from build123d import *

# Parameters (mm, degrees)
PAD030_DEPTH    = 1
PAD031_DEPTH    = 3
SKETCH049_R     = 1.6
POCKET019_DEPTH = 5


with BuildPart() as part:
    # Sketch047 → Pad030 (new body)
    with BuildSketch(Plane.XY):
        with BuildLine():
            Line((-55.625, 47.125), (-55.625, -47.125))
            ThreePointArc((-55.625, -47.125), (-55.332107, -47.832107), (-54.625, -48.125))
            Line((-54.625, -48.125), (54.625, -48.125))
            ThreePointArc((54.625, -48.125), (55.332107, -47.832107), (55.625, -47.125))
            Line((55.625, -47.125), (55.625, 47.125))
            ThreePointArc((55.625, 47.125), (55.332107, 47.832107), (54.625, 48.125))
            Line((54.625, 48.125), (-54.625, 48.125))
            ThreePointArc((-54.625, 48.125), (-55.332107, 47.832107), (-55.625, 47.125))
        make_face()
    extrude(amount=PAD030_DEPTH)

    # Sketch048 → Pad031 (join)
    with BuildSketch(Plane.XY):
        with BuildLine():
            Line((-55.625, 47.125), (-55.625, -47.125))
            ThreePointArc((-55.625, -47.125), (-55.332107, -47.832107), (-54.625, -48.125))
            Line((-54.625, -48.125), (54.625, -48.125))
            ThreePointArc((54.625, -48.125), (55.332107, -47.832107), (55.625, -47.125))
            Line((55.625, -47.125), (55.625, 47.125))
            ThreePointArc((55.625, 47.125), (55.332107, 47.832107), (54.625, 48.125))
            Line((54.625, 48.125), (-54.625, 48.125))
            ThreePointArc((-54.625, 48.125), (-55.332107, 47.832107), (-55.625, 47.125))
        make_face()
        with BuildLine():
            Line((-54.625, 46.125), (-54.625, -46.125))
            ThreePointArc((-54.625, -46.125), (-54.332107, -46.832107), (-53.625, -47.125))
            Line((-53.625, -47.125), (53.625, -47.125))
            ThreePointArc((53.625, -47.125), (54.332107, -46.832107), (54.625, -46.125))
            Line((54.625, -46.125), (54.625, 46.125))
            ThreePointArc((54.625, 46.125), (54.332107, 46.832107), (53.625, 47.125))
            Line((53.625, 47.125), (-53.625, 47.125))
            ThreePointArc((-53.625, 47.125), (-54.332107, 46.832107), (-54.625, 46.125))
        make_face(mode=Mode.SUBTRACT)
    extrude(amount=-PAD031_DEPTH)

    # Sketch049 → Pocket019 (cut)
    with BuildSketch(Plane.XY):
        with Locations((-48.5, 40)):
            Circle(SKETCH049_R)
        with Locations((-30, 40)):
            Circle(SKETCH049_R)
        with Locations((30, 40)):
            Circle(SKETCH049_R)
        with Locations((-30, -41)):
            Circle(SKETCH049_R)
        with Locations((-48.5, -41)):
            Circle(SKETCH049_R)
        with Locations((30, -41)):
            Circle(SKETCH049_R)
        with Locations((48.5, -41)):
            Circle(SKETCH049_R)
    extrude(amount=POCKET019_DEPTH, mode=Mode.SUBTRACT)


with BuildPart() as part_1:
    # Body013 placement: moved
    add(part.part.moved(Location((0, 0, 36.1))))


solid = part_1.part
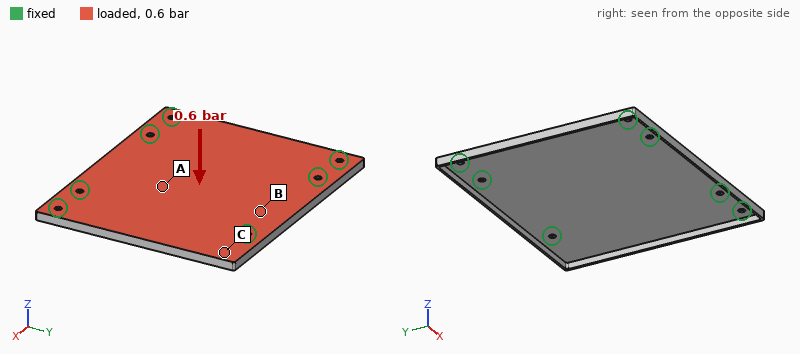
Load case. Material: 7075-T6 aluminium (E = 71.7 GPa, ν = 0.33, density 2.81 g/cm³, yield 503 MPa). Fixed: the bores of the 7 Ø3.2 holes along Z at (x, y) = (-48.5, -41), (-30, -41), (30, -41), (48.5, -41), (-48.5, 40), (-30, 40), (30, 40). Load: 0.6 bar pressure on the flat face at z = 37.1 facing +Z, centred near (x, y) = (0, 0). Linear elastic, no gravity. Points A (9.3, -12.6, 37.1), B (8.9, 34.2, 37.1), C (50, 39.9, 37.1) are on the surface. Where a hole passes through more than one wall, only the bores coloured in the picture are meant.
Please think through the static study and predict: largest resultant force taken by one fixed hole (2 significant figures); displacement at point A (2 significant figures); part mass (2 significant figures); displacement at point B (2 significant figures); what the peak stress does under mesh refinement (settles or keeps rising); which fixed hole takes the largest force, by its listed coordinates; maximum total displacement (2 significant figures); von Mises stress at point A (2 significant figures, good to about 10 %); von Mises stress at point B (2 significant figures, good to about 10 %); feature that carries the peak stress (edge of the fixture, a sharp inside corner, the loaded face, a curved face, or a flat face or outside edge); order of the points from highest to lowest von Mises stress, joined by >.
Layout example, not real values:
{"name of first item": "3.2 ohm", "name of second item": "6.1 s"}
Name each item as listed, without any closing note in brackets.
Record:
{"largest resultant force taken by one fixed hole": "180 N", "displacement at point A": "1.3 mm", "part mass": "33 g", "displacement at point B": "0.46 mm", "what the peak stress does under mesh refinement": "keeps rising", "which fixed hole takes the largest force, by its listed coordinates": "(30, 40)", "maximum total displacement": "1.5 mm", "von Mises stress at point A": "82 MPa", "von Mises stress at point B": "48 MPa", "feature that carries the peak stress": "edge of the fixture", "order of the points from highest to lowest von Mises stress, joined by >": "A > B > C"}
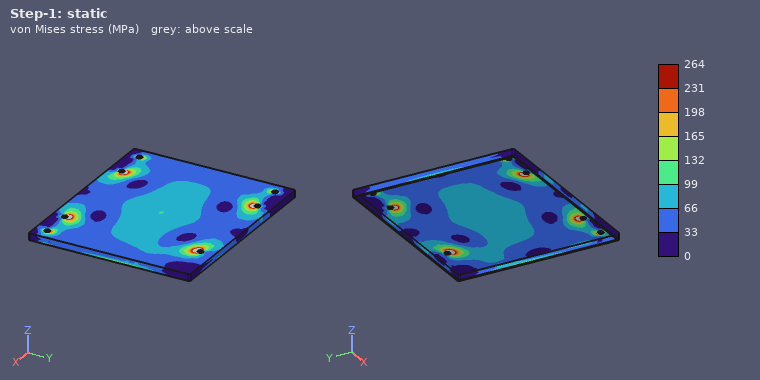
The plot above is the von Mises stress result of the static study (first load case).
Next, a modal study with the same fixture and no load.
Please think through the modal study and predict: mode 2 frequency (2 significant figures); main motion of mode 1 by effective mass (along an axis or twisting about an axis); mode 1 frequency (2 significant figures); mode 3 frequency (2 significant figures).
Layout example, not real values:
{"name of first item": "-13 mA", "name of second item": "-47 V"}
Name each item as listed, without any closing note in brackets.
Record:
{"mode 2 frequency": "1100 Hz", "main motion of mode 1 by effective mass": "along Z", "mode 1 frequency": "740 Hz", "mode 3 frequency": "1400 Hz"}
